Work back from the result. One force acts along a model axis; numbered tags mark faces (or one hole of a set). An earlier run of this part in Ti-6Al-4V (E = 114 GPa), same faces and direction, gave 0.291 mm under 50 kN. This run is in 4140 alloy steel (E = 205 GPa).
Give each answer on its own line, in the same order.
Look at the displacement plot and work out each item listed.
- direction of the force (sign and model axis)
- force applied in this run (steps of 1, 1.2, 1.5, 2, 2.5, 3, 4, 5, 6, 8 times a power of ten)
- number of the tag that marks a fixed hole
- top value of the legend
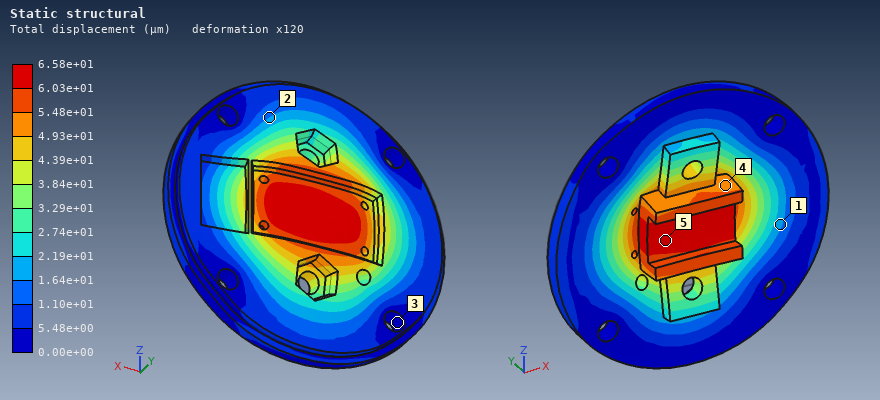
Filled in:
+Y
20 kN
3
6.58e+01 µm
